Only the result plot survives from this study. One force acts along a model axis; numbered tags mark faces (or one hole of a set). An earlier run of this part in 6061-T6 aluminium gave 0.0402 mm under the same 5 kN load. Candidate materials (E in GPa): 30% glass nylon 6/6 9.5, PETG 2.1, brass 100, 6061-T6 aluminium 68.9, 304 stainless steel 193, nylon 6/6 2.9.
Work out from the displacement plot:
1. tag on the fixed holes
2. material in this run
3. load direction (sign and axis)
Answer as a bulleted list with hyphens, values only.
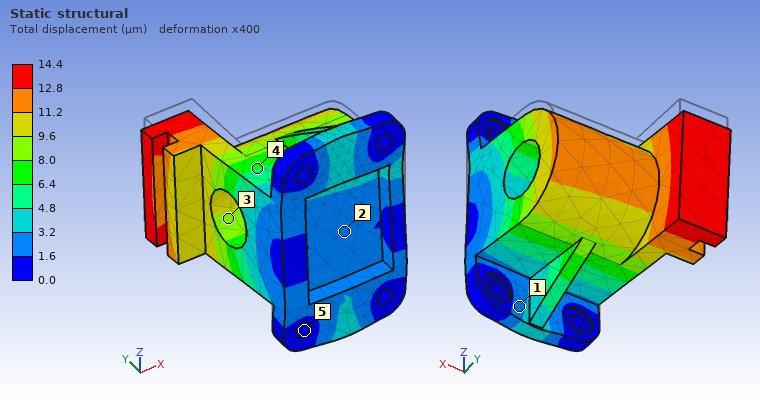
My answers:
- 5
- 304 stainless steel
- -Z
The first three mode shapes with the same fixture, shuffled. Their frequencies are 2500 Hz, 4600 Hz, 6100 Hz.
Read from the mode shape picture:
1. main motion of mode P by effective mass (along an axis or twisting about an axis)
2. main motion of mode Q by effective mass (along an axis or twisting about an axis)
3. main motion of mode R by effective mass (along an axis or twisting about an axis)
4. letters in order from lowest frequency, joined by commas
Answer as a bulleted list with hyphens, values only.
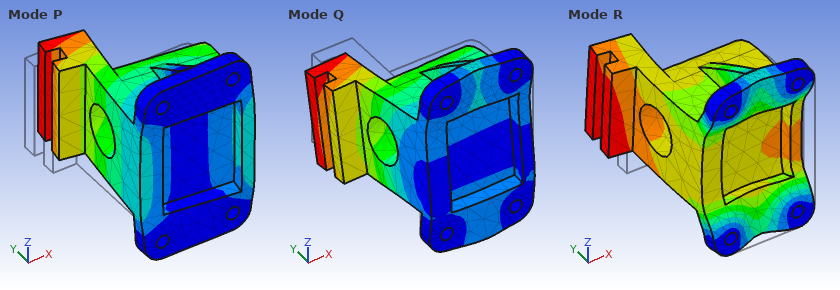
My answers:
- along X
- along Z
- along Y
- P, Q, R
